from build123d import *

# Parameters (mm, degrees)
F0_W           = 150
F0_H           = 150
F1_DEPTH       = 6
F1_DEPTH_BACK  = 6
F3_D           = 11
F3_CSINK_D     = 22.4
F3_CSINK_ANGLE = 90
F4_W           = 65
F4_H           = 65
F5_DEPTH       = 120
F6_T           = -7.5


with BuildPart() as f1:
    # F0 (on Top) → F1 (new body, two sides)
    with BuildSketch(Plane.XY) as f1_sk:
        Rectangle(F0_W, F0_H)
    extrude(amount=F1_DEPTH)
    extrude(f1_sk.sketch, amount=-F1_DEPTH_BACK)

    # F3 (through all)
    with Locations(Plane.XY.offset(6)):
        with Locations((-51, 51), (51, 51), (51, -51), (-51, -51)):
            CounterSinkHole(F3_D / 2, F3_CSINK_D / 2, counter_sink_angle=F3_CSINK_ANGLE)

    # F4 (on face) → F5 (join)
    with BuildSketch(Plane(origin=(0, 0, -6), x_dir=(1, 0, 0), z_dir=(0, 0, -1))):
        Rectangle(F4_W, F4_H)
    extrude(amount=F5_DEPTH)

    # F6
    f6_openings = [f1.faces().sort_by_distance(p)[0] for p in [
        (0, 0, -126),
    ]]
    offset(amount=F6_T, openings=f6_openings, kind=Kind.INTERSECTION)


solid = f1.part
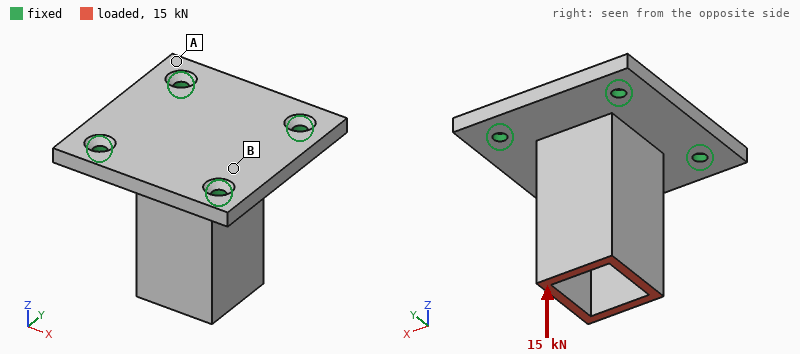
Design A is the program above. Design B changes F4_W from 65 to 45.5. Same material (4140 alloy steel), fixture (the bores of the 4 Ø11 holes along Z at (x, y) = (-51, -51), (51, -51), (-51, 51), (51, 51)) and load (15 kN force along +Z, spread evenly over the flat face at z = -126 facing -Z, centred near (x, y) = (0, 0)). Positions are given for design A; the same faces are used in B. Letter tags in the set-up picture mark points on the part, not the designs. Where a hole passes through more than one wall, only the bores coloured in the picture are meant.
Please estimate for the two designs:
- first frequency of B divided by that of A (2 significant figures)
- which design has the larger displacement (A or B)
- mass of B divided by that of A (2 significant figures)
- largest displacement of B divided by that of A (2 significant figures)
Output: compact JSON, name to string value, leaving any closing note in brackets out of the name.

{"first frequency of B divided by that of A": "0.84", "which design has the larger displacement": "B", "mass of B divided by that of A": "0.93", "largest displacement of B divided by that of A": "1.3"}
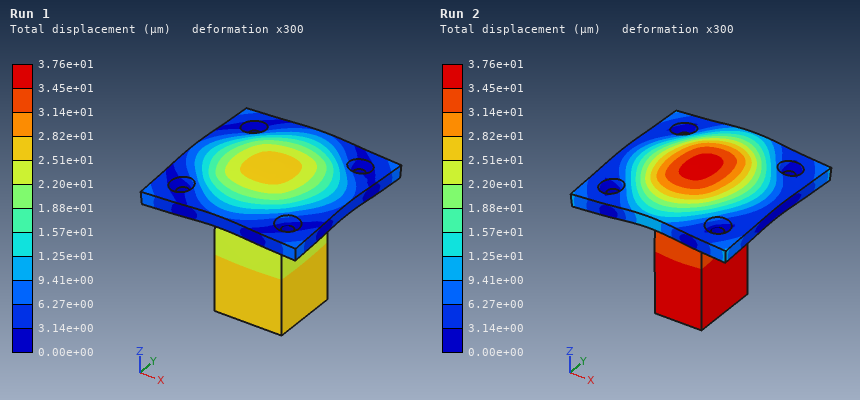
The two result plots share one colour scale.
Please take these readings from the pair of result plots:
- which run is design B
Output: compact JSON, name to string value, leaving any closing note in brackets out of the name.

{"which run is design B": "Run 2"}
